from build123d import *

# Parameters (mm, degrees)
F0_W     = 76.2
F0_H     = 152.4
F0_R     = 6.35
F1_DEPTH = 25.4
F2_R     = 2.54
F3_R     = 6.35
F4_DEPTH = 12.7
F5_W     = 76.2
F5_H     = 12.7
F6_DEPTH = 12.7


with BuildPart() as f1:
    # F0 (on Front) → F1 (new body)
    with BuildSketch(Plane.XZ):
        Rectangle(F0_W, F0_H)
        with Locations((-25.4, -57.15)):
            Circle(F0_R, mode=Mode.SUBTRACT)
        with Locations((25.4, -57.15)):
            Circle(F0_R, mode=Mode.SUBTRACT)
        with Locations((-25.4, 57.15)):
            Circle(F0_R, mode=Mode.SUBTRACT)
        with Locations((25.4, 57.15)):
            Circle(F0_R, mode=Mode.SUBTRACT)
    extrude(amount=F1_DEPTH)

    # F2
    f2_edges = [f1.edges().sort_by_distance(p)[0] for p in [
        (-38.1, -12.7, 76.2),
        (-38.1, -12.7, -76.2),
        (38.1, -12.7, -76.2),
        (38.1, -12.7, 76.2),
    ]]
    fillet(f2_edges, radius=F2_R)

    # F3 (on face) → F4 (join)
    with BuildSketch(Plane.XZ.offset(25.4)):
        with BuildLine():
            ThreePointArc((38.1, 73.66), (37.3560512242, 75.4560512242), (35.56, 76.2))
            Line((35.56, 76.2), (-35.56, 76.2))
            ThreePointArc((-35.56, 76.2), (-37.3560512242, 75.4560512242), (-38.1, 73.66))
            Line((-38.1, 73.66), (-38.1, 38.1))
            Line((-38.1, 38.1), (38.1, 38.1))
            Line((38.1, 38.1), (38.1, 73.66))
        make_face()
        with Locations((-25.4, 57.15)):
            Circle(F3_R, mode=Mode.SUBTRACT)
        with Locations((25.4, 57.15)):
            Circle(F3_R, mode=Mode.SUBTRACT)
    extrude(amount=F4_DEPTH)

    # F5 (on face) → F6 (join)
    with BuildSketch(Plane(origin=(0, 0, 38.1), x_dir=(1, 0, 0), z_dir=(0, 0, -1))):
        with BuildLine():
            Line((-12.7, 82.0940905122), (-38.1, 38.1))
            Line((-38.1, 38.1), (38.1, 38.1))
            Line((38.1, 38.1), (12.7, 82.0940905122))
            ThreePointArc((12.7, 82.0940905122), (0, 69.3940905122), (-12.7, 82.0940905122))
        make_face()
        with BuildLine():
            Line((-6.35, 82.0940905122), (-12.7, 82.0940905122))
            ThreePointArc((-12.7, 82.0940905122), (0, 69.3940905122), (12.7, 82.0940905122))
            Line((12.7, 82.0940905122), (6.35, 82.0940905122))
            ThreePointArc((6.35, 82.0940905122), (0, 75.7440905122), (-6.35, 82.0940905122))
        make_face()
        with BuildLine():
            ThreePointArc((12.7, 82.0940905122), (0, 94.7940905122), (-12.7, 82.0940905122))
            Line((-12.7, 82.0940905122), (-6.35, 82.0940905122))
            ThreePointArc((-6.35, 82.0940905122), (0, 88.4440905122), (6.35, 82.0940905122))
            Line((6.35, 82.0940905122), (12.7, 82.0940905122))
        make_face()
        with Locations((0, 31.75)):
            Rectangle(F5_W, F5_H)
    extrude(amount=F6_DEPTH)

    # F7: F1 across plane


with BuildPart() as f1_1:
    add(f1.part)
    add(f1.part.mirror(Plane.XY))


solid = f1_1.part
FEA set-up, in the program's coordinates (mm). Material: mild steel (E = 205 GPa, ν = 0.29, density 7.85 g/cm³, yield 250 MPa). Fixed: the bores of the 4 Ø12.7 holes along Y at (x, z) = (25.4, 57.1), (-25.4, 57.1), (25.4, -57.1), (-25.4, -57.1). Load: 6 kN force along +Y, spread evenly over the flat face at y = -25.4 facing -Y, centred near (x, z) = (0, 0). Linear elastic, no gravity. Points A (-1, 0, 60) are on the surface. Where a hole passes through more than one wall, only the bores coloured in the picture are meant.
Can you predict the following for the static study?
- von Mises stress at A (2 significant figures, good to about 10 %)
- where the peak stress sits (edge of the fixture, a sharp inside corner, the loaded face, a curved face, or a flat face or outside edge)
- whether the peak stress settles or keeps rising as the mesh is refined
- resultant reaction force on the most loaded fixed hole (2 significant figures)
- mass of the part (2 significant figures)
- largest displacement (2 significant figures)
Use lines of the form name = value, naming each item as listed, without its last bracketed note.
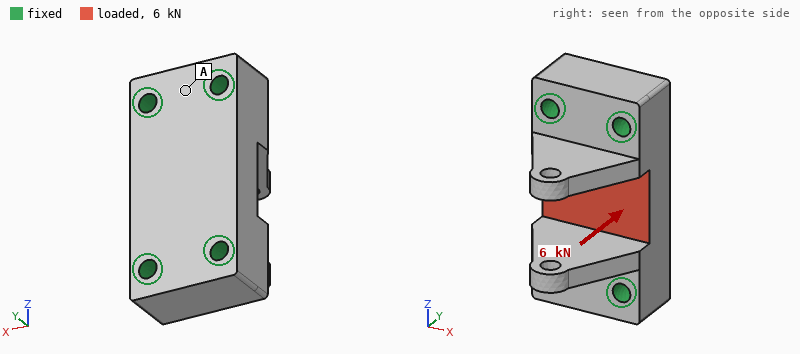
von Mises stress at A = 1.3 MPa
where the peak stress sits = edge of the fixture
whether the peak stress settles or keeps rising as the mesh is refined = keeps rising
resultant reaction force on the most loaded fixed hole = 1.6 kN
mass of the part = 3.4 kg
largest displacement = 2.1 µm
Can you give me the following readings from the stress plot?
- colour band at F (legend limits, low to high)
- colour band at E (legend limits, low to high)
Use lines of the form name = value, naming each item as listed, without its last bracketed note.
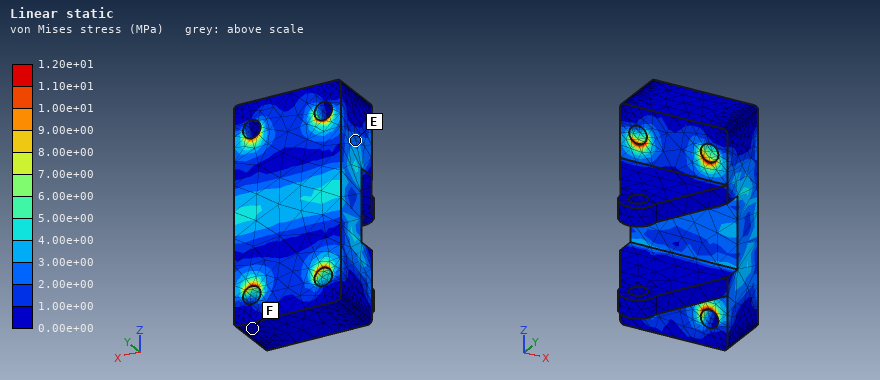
colour band at F = 0.00e+00 to 1.00e+00 MPa
colour band at E = 2.00e+00 to 3.00e+00 MPa
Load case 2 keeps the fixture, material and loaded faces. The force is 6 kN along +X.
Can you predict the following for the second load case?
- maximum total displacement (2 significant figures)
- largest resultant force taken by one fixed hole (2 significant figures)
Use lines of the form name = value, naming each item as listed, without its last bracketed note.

maximum total displacement = 1.6 µm
largest resultant force taken by one fixed hole = 2.0 kN
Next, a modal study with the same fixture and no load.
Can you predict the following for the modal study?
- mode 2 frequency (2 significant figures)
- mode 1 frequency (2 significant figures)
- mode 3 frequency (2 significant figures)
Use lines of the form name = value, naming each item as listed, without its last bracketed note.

mode 2 frequency = 4200 Hz
mode 1 frequency = 4200 Hz
mode 3 frequency = 9500 Hz
